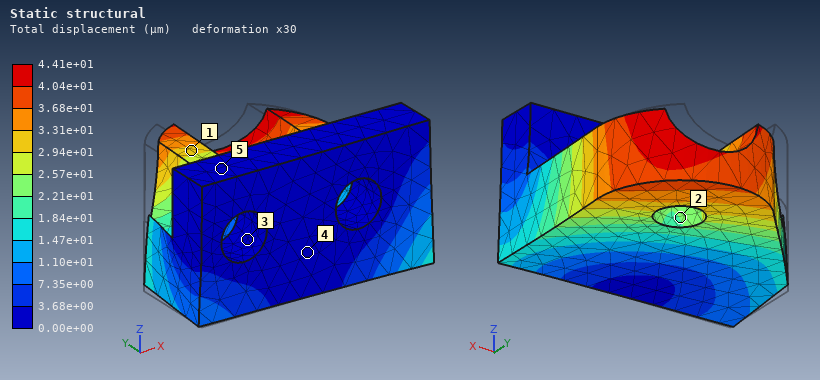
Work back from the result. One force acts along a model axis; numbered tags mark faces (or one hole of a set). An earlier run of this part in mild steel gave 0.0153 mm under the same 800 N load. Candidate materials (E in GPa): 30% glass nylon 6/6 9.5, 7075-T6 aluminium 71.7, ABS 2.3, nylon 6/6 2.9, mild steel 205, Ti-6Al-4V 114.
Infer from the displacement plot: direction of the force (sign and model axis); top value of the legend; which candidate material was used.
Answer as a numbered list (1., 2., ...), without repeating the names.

1. +X
2. 4.41e+01 µm
3. 7075-T6 aluminium
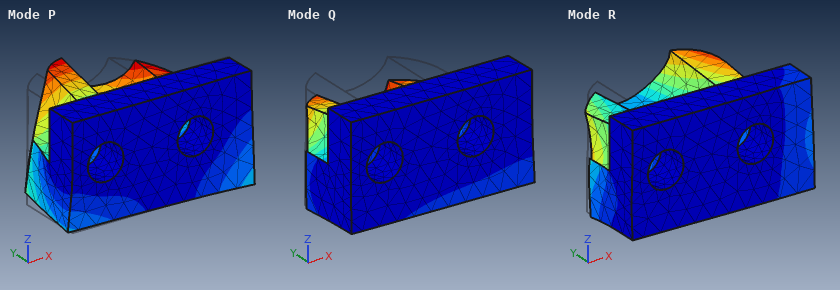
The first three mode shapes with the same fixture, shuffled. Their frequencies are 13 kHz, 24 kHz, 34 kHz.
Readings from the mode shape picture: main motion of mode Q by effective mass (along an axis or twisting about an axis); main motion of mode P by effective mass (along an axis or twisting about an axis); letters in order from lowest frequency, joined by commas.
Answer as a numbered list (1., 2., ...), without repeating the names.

1. along Z
2. along X
3. Q, P, R
